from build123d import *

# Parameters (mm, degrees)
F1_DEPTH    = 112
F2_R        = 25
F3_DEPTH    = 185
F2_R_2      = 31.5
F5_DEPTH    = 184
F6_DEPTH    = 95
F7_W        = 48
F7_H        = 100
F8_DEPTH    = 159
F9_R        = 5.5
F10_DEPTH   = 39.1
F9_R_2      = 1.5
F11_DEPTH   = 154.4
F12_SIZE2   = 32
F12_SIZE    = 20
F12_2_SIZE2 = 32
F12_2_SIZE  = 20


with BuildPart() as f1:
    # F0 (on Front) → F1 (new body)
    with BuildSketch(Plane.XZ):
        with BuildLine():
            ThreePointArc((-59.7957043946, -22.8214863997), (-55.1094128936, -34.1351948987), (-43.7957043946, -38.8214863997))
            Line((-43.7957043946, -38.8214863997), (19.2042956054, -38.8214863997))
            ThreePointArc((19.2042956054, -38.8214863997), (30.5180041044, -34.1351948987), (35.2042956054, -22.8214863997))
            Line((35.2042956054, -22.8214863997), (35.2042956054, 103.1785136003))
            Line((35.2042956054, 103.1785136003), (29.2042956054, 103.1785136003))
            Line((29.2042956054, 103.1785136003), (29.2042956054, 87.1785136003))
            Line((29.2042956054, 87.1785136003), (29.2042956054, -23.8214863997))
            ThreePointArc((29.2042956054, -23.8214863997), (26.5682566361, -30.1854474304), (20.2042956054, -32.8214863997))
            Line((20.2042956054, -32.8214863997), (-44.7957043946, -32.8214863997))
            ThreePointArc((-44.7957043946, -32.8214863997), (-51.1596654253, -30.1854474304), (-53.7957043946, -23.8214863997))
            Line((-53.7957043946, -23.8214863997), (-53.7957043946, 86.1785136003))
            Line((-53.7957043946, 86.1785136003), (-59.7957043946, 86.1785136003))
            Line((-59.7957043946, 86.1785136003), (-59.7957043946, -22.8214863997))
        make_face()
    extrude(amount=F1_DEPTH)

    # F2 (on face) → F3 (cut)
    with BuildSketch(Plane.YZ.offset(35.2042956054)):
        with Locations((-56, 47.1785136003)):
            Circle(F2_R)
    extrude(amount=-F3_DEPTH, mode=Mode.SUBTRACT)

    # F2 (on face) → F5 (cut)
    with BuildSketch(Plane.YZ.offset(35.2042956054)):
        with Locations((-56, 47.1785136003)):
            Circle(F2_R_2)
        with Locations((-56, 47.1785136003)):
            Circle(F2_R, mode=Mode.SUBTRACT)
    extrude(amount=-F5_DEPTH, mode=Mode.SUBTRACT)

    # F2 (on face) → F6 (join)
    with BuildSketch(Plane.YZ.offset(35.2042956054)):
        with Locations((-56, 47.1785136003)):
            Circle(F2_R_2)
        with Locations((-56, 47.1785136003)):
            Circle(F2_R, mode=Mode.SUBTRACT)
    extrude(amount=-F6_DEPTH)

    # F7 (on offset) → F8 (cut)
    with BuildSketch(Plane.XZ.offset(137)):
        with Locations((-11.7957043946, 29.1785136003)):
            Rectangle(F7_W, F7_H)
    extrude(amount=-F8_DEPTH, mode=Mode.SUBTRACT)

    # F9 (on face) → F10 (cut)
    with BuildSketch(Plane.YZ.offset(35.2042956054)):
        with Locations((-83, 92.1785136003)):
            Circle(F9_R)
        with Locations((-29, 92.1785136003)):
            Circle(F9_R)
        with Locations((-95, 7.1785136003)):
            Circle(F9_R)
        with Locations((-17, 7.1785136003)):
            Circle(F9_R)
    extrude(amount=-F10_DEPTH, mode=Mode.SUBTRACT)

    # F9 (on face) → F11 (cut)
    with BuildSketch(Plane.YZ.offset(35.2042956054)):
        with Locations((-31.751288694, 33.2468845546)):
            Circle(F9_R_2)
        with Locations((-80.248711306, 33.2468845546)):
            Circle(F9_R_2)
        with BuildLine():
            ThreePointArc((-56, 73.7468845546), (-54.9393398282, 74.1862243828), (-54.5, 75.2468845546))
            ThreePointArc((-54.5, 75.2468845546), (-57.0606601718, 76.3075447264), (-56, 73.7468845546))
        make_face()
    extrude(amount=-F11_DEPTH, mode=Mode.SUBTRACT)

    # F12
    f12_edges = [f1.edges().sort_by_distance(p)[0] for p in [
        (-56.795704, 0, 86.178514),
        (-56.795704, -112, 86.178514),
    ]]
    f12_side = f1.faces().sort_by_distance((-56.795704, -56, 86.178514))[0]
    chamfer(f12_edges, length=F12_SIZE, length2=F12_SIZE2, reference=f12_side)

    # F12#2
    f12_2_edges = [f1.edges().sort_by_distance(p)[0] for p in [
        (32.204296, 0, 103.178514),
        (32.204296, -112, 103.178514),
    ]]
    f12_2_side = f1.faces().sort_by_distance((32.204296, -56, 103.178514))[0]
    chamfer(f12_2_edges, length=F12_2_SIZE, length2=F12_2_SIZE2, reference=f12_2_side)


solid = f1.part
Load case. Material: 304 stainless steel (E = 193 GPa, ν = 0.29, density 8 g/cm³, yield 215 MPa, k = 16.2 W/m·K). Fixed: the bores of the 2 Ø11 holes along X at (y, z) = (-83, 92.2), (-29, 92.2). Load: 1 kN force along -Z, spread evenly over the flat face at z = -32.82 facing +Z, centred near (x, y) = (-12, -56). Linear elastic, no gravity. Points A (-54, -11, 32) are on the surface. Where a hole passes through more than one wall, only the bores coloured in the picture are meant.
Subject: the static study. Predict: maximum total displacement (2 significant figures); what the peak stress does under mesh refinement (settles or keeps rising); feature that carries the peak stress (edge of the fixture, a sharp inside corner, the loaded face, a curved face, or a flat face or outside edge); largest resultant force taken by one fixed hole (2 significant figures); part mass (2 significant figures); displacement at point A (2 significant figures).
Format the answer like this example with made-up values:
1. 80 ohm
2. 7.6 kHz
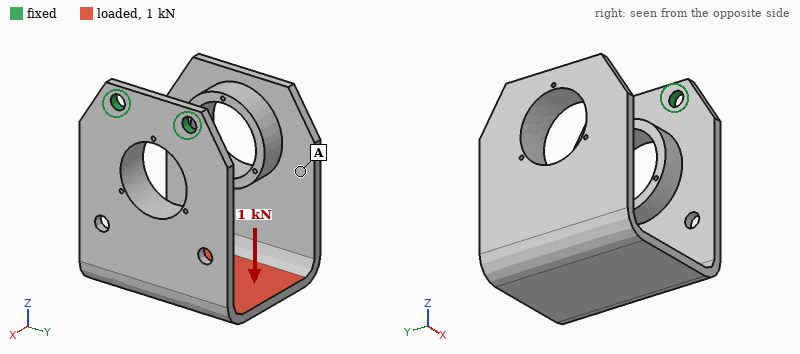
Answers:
1. 1.6 mm
2. keeps rising
3. edge of the fixture
4. 560 N
5. 1.9 kg
6. 1.2 mm
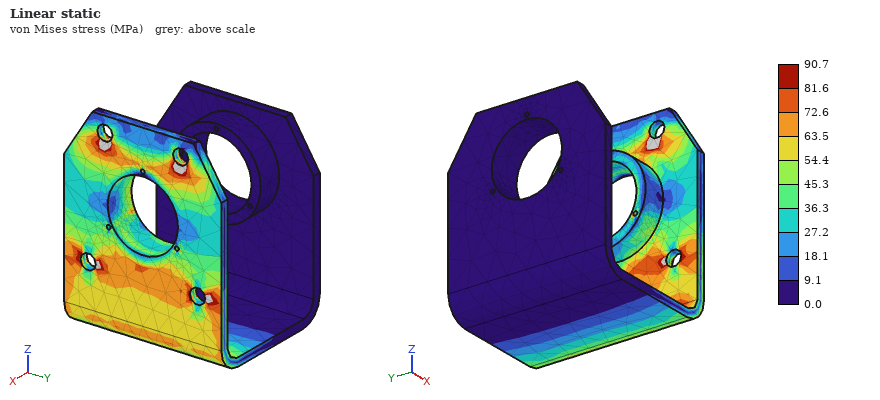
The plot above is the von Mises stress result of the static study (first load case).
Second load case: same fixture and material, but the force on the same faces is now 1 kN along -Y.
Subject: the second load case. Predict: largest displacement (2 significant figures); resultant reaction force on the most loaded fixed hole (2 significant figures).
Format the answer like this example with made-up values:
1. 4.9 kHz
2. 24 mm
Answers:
1. 0.64 mm
2. 2.2 kN
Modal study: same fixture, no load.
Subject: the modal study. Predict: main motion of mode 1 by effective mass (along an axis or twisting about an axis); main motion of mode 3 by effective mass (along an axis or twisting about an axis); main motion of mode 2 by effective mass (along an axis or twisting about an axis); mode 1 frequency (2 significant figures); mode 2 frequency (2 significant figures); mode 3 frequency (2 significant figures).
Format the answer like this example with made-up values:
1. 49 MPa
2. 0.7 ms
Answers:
1. along Z
2. along X
3. along Y
4. 95 Hz
5. 140 Hz
6. 150 Hz
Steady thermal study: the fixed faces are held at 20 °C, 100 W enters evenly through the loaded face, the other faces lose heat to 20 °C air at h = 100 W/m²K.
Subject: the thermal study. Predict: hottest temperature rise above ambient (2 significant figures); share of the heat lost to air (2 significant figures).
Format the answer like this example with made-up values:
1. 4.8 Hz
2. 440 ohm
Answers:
1. 83 K
2. 100 %
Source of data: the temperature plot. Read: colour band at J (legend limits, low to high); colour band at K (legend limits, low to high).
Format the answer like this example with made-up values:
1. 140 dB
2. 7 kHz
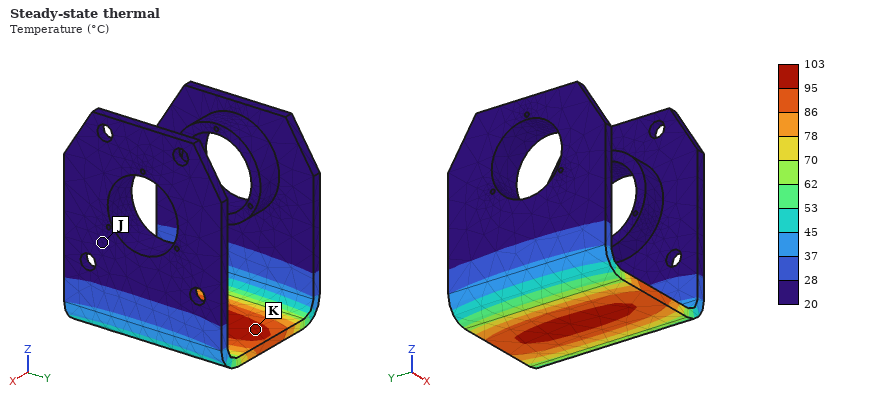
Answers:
1. 20 to 28 °C
2. 95 to 103 °C
